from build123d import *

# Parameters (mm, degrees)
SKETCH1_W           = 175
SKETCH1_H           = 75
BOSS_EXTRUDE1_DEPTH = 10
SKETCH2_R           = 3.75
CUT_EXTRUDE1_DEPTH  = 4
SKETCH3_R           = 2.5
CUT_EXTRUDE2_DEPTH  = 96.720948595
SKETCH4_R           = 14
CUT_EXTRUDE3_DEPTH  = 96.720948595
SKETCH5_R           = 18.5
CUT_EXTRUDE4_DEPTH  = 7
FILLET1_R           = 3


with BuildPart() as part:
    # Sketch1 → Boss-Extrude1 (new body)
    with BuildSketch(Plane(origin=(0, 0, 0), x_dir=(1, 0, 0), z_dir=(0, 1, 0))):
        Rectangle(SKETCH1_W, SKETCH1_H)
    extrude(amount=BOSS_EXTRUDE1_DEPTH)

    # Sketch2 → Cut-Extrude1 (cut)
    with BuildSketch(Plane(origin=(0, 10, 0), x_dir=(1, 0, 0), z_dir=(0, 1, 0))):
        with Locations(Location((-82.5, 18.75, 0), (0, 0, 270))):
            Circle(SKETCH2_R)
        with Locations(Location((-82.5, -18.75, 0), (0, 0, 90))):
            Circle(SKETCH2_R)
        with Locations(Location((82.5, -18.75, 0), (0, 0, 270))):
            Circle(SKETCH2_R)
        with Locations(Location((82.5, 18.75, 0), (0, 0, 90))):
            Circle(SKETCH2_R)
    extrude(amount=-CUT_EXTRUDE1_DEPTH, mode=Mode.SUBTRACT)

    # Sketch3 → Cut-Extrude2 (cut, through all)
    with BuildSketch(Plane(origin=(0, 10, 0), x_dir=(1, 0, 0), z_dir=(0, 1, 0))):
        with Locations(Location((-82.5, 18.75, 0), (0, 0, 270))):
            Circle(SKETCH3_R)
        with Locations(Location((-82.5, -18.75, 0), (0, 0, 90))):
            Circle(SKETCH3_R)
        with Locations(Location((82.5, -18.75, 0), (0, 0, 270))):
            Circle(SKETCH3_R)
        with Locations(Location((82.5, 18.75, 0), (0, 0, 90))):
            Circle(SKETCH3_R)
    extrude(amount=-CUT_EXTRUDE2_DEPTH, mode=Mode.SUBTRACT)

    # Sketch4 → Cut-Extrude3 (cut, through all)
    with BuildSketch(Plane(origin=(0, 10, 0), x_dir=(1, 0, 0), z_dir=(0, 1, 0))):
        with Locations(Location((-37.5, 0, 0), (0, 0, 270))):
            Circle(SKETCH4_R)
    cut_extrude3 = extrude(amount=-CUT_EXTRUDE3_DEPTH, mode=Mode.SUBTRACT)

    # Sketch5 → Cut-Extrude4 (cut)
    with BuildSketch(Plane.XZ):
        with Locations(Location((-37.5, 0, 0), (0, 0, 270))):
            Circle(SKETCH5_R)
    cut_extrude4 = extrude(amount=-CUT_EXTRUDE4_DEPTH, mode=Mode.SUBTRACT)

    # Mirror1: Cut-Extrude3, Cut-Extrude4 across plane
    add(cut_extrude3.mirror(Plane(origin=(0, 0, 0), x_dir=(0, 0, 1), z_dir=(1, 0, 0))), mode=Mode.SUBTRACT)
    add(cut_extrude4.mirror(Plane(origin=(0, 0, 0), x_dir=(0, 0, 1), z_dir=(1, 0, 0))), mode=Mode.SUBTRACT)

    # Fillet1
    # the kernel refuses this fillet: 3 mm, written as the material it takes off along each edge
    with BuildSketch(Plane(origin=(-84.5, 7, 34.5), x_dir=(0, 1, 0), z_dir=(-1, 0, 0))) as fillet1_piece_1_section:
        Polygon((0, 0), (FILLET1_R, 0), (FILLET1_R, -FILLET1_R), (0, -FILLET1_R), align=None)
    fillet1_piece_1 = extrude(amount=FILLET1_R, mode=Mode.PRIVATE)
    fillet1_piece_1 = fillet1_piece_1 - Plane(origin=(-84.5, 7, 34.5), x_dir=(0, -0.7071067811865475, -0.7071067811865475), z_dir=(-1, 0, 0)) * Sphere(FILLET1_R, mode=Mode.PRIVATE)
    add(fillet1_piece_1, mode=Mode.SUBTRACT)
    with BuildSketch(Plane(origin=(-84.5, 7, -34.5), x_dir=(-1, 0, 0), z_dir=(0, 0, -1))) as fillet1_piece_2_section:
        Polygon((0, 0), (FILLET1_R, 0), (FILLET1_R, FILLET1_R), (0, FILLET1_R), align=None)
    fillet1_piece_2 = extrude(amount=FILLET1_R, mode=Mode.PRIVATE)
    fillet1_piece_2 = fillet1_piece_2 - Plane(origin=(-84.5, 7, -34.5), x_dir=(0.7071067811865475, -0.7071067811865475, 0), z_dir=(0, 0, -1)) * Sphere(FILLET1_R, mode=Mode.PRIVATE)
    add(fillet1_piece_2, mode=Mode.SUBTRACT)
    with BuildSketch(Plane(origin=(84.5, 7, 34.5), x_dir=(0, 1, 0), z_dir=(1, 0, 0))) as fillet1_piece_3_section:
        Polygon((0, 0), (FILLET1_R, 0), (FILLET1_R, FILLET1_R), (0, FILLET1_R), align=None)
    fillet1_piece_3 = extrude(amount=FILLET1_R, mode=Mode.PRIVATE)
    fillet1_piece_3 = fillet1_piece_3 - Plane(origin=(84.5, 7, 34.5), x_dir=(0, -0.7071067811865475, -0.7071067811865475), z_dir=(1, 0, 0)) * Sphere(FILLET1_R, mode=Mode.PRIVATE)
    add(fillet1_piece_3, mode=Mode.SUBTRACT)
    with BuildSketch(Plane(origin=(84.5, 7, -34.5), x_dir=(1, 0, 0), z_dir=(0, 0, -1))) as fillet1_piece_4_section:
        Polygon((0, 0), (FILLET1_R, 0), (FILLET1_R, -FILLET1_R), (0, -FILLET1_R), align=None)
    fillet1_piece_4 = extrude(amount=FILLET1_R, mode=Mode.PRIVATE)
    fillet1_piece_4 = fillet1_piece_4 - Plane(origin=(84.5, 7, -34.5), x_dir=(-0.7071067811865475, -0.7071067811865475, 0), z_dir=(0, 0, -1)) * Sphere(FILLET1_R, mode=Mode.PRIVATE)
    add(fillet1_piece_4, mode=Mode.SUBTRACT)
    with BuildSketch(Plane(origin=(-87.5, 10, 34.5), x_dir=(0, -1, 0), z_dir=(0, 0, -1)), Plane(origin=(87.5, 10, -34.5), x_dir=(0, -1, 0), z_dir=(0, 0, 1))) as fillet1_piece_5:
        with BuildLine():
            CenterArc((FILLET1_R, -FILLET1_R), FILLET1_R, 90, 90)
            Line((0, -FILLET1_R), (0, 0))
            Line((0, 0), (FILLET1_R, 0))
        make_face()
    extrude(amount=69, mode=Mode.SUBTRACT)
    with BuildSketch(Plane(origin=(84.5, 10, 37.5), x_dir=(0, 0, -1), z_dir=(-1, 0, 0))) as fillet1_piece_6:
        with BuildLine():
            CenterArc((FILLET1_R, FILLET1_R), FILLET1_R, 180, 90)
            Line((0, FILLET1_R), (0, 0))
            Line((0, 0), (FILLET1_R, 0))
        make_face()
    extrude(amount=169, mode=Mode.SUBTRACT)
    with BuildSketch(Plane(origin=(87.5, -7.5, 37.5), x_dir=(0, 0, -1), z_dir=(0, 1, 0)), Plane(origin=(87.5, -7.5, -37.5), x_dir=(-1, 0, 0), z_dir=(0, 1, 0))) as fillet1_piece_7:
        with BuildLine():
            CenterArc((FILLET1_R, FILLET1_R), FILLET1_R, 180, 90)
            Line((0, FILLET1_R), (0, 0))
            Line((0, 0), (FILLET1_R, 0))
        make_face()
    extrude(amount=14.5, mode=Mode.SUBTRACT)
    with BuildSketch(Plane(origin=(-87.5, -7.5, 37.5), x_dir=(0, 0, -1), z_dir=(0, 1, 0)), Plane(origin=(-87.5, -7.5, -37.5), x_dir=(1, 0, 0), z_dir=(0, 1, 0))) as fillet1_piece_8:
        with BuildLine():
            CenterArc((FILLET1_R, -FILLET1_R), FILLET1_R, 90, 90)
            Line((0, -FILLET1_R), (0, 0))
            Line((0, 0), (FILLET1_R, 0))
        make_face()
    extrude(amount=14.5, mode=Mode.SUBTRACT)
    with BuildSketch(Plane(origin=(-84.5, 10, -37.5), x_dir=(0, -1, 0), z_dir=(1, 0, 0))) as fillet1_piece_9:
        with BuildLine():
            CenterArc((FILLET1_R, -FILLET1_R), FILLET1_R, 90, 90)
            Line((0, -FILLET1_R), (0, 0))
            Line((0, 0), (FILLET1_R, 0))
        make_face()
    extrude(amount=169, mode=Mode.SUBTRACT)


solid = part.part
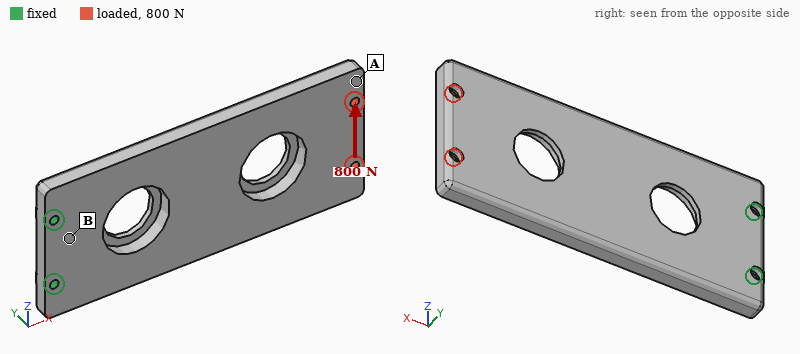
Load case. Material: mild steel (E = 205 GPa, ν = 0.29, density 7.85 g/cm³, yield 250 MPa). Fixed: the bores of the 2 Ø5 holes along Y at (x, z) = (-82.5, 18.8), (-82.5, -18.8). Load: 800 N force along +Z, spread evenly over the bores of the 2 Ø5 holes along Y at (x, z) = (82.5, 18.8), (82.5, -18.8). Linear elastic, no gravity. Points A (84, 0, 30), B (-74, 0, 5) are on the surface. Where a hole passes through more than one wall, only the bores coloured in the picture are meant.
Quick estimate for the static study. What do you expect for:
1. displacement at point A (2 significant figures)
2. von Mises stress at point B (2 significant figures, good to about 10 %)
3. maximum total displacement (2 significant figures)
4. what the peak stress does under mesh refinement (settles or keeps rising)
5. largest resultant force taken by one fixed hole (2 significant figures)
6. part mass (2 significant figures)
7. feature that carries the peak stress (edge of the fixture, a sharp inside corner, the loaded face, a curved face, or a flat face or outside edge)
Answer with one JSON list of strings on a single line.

["44 µm", "16 MPa", "46 µm", "keeps rising", "3.3 kN", "870 g", "edge of the fixture"]
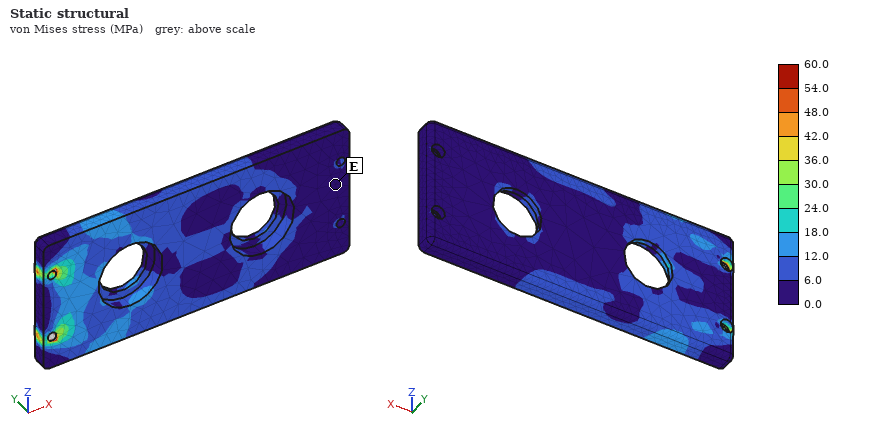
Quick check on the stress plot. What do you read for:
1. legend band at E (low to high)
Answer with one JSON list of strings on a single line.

["0.0 to 6.0 MPa"]
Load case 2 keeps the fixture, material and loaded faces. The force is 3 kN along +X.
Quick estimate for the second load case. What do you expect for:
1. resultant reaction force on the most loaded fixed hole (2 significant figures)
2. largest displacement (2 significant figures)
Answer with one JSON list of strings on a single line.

["1.5 kN", "0.10 mm"]
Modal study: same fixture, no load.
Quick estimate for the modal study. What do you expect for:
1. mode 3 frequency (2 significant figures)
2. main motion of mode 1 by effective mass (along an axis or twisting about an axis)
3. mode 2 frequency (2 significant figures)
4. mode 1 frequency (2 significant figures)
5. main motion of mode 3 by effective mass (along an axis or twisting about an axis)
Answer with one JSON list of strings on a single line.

["1400 Hz", "along Y", "1100 Hz", "230 Hz", "along Z"]
